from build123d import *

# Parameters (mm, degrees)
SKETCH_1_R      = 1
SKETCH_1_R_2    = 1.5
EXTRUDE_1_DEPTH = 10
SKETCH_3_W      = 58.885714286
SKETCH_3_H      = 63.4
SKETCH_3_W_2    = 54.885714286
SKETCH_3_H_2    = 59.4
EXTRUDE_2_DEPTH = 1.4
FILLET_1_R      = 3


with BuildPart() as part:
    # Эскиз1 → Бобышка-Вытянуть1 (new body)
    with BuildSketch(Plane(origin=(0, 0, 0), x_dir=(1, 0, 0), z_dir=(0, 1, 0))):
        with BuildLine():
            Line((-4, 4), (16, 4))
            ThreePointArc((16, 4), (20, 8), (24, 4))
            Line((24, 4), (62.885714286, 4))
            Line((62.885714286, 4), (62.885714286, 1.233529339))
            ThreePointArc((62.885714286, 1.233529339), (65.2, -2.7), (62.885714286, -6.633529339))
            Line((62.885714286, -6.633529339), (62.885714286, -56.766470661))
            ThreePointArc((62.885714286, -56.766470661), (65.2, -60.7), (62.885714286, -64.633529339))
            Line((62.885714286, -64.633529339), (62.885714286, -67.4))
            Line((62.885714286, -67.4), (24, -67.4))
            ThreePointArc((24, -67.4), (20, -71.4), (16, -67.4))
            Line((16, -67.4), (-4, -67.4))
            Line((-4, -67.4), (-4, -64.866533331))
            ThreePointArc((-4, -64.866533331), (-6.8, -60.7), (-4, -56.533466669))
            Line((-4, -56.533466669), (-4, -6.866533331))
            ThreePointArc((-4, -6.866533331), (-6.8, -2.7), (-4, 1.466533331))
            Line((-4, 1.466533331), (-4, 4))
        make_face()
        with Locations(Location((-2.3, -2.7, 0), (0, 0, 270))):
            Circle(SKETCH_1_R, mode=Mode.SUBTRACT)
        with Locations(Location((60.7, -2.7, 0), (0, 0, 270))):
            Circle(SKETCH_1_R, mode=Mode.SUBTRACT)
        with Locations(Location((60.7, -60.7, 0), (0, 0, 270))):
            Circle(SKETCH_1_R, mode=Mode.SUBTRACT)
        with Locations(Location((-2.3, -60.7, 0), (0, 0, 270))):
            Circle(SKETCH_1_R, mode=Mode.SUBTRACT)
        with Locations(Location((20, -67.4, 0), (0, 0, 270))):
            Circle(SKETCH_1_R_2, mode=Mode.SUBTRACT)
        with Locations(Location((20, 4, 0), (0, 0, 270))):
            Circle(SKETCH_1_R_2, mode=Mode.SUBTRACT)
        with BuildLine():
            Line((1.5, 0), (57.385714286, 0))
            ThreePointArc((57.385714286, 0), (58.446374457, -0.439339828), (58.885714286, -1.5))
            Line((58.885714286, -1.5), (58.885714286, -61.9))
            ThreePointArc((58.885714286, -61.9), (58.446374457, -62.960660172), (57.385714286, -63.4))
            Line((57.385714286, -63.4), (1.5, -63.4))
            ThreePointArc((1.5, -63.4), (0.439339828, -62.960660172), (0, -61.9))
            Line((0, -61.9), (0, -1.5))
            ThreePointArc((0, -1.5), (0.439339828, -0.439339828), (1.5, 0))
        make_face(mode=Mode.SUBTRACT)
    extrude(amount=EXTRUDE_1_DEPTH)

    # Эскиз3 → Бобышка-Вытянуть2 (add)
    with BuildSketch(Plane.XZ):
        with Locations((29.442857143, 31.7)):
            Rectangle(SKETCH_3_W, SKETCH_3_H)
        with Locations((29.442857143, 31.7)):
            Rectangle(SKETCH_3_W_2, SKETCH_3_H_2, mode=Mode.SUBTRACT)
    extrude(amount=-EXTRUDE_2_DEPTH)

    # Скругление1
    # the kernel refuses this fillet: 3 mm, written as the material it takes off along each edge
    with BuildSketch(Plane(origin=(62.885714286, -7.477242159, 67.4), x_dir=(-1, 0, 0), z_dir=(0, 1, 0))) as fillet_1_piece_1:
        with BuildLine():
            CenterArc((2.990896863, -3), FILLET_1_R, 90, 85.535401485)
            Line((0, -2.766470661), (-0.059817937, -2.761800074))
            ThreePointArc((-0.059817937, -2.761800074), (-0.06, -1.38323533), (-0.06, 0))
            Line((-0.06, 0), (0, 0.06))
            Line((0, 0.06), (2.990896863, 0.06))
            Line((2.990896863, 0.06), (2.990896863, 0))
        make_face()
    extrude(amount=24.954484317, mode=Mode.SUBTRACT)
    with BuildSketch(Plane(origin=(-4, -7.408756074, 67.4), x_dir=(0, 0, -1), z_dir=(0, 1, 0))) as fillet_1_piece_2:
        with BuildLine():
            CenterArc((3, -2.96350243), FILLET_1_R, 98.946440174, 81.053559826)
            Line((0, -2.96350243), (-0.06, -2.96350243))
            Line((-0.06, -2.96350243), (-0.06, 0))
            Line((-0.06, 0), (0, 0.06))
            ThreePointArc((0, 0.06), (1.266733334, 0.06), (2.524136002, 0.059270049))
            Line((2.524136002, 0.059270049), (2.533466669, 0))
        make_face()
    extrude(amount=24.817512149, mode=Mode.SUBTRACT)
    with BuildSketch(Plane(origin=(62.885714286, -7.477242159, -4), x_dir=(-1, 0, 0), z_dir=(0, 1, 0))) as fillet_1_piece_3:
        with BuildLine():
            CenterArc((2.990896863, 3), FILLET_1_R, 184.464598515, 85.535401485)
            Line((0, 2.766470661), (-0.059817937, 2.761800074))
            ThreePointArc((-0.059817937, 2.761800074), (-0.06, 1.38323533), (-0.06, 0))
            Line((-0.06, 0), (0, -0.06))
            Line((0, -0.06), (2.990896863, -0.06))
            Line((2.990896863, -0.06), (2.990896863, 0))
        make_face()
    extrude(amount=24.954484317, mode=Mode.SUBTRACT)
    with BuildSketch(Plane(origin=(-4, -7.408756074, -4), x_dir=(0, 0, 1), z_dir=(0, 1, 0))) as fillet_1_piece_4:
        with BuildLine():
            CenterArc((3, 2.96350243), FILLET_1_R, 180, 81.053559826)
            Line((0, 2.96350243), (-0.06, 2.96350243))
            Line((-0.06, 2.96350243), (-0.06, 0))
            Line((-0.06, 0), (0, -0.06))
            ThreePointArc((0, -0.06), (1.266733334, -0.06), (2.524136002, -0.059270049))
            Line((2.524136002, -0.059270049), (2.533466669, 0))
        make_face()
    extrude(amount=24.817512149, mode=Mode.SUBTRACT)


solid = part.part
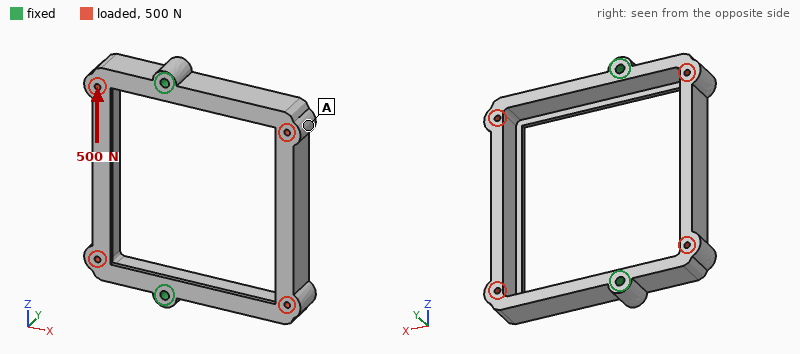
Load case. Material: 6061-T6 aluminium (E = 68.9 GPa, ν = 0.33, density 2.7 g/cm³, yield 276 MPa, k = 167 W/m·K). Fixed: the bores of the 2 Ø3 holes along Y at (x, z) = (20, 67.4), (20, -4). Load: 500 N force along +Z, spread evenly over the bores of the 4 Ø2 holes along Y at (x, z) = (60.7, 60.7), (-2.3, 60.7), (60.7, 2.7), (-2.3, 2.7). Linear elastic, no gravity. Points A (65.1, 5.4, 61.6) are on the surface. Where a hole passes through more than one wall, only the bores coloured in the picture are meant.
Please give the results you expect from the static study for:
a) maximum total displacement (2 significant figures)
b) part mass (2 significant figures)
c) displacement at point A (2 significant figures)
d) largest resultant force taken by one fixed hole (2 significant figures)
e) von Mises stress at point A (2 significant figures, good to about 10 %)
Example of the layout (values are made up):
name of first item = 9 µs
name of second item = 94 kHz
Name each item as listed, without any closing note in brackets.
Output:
maximum total displacement = 0.19 mm
part mass = 32 g
displacement at point A = 0.19 mm
largest resultant force taken by one fixed hole = 250 N
von Mises stress at point A = 13 MPa
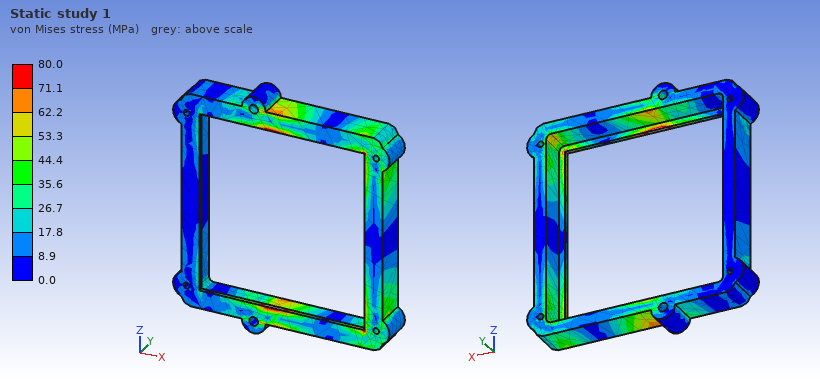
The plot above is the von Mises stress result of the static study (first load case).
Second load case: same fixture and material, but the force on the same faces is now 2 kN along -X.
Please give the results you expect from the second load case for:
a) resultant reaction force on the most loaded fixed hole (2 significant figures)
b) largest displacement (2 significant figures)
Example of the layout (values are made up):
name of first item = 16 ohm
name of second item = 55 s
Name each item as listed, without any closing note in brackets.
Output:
resultant reaction force on the most loaded fixed hole = 1.0 kN
largest displacement = 70 µm
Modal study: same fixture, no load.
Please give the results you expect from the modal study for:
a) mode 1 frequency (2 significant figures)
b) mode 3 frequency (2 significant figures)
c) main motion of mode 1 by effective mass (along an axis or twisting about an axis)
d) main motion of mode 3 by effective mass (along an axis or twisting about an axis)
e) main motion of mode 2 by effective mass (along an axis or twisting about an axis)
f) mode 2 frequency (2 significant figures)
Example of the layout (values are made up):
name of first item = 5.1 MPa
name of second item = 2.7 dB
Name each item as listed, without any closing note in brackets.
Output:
mode 1 frequency = 1800 Hz
mode 3 frequency = 3600 Hz
main motion of mode 1 by effective mass = along Z
main motion of mode 3 by effective mass = twisting about X
main motion of mode 2 by effective mass = along Y
mode 2 frequency = 2200 Hz
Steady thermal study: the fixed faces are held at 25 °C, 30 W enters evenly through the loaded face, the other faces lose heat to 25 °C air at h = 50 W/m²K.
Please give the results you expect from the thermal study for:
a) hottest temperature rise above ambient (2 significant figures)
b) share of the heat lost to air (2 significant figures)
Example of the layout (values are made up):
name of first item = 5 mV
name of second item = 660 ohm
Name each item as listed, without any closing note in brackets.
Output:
hottest temperature rise above ambient = 32 K
share of the heat lost to air = 25 %
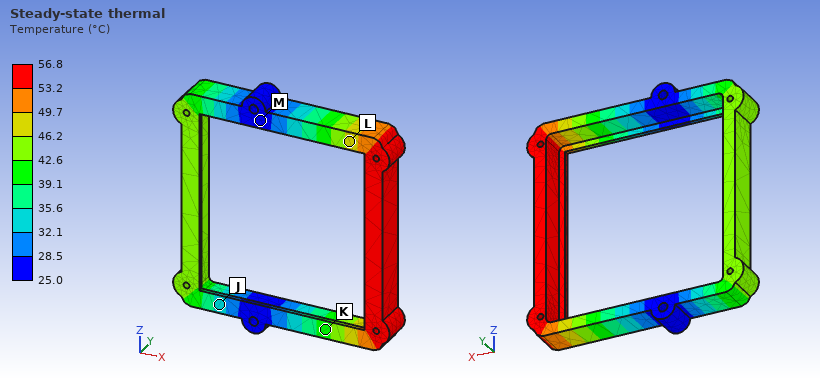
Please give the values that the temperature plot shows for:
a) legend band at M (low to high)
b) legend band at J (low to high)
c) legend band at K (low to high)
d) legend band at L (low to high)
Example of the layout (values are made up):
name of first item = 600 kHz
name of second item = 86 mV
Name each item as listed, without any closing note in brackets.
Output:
legend band at M = 25.0 to 28.5 °C
legend band at J = 32.1 to 35.6 °C
legend band at K = 39.1 to 42.6 °C
legend band at L = 46.2 to 49.7 °C
